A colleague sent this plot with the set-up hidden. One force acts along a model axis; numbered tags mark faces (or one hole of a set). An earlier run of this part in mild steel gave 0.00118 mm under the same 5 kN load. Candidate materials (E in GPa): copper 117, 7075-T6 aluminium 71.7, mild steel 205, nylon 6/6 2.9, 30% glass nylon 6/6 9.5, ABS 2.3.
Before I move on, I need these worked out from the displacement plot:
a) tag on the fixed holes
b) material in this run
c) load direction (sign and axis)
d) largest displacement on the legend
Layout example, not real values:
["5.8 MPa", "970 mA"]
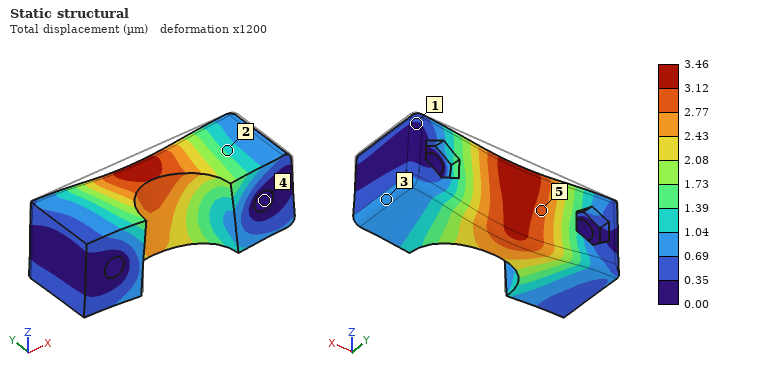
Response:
["4", "7075-T6 aluminium", "-Z", "3.46 µm"]
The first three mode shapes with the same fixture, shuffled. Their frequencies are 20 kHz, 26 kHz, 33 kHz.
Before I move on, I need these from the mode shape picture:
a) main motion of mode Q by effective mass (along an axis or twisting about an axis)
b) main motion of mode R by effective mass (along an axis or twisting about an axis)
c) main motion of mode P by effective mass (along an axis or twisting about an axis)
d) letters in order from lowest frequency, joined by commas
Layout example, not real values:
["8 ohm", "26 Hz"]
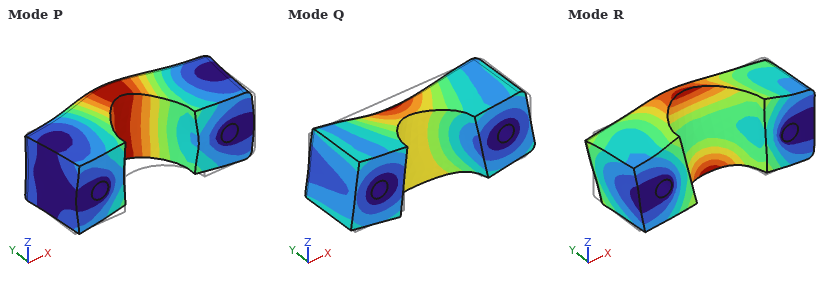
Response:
["along Z", "twisting about X", "along Y", "Q, P, R"]
